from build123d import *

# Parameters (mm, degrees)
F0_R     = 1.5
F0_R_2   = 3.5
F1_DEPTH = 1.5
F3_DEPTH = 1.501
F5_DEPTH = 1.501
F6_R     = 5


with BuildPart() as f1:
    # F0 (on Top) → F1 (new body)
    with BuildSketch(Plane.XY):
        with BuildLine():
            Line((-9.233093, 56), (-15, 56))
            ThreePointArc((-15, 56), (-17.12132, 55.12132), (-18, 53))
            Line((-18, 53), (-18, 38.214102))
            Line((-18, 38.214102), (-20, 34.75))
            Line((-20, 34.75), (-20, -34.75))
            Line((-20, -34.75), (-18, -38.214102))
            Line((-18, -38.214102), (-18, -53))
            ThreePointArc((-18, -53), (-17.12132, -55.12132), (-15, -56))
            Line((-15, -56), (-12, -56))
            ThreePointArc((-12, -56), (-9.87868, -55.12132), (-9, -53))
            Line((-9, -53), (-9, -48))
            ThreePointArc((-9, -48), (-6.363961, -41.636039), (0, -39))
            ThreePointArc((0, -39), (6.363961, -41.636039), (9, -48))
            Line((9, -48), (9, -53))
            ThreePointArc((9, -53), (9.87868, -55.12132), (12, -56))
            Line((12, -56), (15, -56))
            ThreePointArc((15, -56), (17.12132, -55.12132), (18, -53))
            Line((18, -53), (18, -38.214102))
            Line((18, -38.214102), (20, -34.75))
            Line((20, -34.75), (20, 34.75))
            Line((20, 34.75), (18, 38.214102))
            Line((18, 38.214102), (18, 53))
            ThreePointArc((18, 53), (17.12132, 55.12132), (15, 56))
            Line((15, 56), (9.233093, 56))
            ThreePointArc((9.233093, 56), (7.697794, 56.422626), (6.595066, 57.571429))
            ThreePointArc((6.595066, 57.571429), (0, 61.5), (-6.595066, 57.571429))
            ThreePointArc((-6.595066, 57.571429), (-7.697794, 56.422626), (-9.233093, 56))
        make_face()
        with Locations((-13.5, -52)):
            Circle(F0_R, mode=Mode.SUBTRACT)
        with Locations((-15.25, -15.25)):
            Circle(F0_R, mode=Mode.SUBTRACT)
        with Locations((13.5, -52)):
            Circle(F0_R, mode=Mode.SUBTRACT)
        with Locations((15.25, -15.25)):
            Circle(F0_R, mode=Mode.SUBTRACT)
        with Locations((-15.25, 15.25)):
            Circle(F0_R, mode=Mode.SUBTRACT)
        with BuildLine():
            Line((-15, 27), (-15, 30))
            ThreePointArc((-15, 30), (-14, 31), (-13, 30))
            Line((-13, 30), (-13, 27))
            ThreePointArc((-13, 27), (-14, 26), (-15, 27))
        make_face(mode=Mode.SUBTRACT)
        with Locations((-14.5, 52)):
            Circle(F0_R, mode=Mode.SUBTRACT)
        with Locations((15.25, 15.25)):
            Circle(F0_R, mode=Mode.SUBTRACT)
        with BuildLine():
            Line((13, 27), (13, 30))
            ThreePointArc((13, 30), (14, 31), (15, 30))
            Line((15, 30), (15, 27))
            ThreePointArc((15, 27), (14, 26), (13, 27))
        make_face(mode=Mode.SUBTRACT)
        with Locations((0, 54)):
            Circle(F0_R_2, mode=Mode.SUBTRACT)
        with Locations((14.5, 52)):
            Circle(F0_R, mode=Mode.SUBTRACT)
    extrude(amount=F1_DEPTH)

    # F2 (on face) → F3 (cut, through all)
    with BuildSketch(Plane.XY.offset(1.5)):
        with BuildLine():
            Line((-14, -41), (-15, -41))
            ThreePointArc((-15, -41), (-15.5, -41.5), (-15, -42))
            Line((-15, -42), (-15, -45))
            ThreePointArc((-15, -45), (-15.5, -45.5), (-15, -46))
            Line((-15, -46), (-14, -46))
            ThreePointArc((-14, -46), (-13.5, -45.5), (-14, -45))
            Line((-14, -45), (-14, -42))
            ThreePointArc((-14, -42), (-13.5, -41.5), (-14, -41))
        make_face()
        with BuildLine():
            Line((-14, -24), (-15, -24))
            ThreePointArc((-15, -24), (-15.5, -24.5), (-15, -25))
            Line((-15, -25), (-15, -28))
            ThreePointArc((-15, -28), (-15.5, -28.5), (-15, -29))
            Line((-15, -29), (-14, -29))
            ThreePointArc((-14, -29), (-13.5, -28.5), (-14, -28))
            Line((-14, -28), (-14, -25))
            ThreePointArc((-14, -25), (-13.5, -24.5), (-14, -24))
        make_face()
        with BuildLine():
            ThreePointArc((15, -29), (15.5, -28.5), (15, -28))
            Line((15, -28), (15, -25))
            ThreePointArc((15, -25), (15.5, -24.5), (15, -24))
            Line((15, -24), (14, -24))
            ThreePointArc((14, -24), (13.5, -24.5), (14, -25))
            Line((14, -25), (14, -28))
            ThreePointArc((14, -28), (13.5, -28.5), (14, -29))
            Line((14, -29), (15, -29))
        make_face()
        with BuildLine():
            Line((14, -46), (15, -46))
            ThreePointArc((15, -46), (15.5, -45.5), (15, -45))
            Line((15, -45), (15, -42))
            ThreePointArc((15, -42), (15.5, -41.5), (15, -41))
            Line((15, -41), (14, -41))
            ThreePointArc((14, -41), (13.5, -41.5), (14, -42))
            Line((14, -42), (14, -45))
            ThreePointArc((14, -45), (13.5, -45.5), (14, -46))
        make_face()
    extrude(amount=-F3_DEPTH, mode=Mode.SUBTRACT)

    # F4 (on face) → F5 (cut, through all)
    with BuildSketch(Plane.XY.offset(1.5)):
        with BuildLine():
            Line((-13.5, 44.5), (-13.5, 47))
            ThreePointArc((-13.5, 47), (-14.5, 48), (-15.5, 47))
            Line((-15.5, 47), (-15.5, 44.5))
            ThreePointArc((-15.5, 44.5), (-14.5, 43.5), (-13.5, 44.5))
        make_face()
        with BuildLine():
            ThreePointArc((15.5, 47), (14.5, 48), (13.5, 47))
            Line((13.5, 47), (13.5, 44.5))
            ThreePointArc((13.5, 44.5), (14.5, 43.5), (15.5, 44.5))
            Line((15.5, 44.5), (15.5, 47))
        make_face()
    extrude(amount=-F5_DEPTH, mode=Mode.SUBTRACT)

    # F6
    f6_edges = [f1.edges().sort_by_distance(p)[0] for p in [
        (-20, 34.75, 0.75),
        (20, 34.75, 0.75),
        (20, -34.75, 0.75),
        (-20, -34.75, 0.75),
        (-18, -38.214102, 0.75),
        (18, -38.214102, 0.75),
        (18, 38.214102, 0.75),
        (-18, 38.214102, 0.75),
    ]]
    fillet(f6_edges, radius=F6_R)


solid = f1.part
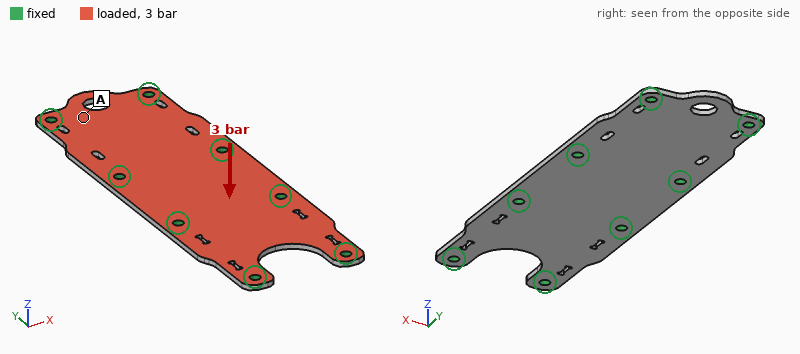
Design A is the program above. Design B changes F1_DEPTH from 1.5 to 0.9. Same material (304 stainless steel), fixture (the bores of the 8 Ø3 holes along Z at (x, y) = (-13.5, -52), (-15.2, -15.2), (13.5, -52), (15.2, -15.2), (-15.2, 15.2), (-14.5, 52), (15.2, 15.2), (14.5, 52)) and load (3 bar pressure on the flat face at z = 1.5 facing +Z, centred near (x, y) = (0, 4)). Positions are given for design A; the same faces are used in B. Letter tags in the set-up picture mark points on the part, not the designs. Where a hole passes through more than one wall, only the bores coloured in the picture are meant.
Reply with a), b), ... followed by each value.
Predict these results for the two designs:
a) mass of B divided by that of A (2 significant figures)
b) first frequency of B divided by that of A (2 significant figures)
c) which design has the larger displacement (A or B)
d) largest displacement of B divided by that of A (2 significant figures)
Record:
a) 0.60
b) 0.61
c) B
d) 4.5
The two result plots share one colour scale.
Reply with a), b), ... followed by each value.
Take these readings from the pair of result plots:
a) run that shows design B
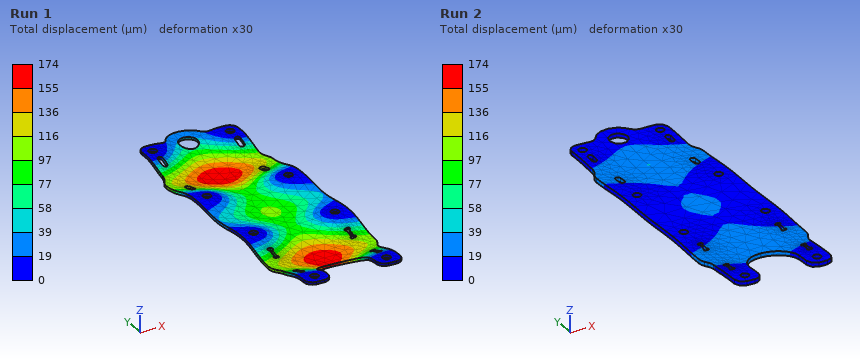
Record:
a) Run 1
